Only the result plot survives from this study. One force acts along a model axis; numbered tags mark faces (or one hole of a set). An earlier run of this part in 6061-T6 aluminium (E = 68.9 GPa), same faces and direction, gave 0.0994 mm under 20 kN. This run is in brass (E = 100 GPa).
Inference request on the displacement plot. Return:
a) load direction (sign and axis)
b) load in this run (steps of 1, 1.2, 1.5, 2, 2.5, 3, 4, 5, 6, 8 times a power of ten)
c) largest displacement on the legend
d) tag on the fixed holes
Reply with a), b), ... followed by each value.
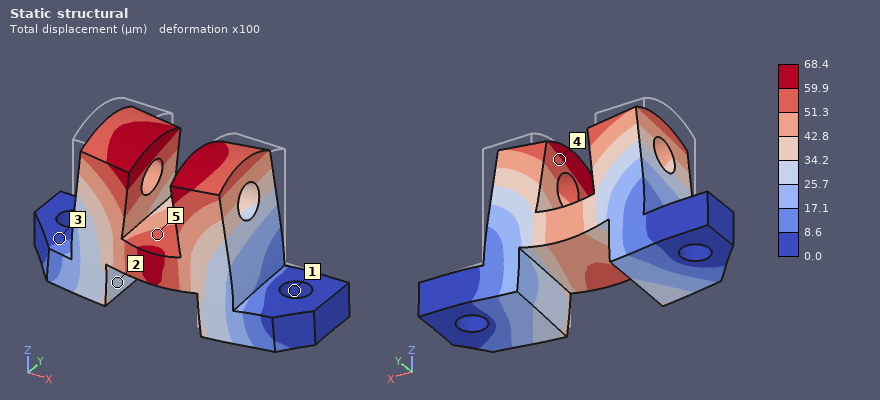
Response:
a) -Z
b) 20 kN
c) 68.4 µm
d) 1
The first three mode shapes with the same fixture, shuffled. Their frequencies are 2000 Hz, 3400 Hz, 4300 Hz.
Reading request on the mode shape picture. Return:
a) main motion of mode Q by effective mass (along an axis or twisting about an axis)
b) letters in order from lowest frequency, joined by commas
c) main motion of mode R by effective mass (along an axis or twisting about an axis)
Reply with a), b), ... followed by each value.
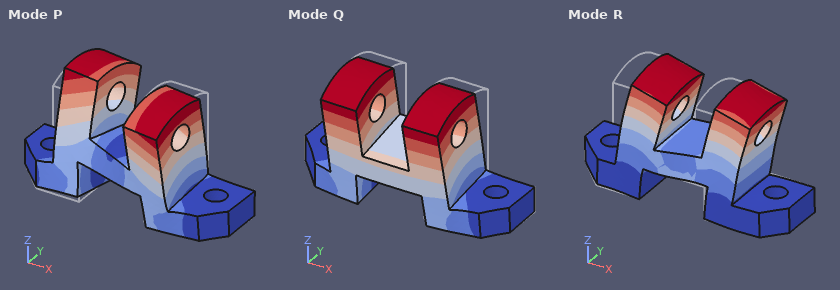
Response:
a) along Y
b) Q, P, R
c) along X
